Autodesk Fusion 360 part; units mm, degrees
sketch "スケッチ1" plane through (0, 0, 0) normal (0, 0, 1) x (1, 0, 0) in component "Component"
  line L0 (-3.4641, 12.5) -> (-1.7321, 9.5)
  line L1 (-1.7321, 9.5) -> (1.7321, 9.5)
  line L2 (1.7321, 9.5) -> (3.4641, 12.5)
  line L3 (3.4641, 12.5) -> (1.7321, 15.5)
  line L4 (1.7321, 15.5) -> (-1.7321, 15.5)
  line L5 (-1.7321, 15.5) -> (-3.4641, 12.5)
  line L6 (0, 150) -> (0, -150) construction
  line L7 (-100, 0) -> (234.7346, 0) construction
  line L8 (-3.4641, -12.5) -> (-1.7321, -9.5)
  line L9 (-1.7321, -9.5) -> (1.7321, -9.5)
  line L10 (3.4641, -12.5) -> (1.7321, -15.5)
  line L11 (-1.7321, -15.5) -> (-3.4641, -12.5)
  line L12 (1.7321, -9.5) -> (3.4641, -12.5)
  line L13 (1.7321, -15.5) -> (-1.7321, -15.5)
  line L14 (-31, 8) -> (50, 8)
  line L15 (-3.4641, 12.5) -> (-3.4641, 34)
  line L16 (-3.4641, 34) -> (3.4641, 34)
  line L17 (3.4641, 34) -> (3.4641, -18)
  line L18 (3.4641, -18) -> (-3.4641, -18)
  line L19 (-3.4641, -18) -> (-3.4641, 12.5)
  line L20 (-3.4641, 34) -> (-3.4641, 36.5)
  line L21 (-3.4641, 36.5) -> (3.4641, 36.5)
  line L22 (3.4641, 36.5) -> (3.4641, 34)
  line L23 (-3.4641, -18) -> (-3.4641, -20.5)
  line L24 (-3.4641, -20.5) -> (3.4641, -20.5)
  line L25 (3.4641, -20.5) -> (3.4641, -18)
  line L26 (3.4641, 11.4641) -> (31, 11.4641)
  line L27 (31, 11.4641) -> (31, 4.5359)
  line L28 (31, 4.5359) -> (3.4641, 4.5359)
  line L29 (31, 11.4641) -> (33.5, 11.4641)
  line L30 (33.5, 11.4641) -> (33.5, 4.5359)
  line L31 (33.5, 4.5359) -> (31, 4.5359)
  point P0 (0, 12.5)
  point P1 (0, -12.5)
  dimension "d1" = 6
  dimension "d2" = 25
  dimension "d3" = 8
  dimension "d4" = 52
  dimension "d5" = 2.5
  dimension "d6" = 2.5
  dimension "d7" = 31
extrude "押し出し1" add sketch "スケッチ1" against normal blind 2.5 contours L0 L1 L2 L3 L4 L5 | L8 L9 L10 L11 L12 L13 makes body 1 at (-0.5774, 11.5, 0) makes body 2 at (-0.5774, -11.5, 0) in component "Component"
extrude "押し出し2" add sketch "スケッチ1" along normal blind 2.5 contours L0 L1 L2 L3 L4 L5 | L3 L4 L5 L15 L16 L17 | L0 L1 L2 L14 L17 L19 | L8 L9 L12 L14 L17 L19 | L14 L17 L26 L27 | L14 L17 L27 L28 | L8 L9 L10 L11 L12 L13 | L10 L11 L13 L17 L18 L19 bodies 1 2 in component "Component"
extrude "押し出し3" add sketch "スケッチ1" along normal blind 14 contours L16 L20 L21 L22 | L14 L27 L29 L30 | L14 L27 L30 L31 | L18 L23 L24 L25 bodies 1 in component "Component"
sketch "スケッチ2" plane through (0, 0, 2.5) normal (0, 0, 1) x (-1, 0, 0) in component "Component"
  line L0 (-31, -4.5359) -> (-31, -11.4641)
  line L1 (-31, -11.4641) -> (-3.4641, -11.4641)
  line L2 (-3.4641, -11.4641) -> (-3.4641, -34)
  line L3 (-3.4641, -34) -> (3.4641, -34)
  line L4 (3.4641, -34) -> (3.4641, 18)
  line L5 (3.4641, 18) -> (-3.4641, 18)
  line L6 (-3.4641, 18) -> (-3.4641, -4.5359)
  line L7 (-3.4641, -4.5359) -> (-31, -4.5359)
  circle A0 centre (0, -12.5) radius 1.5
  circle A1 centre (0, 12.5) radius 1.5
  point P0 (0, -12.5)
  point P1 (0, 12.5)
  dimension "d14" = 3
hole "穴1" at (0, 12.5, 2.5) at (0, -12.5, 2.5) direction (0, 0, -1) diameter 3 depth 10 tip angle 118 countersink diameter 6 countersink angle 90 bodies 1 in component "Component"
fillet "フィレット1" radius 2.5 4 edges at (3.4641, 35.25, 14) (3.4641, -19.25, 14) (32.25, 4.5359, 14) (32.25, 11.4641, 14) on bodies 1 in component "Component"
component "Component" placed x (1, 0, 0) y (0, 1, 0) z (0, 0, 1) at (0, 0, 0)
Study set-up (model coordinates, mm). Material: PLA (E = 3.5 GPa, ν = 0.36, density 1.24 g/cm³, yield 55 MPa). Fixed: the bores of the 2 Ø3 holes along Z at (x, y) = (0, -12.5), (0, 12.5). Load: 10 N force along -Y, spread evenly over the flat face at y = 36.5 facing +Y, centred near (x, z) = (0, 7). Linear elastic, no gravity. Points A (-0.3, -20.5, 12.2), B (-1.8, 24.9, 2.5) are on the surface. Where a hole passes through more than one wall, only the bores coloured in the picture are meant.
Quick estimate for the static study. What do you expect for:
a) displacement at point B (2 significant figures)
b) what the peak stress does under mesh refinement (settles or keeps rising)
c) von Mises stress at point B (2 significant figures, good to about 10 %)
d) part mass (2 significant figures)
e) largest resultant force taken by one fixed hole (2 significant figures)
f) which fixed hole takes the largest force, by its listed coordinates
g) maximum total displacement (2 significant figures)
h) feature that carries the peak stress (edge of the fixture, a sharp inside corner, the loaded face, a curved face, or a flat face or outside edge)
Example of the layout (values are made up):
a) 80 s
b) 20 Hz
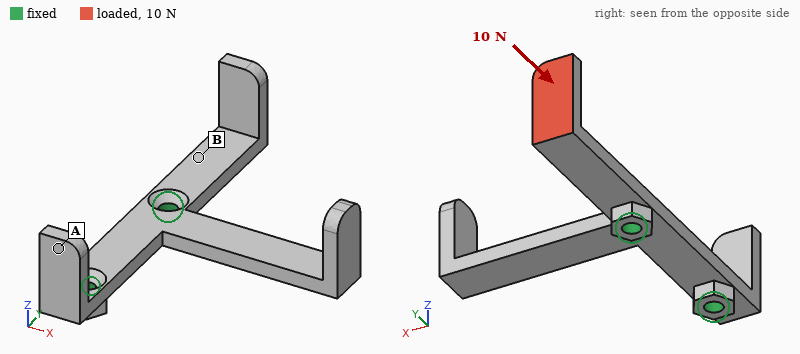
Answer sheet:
a) 0.13 mm
b) keeps rising
c) 8.4 MPa
d) 2.7 g
e) 8.2 N
f) (0, 12.5)
g) 0.75 mm
h) edge of the fixture
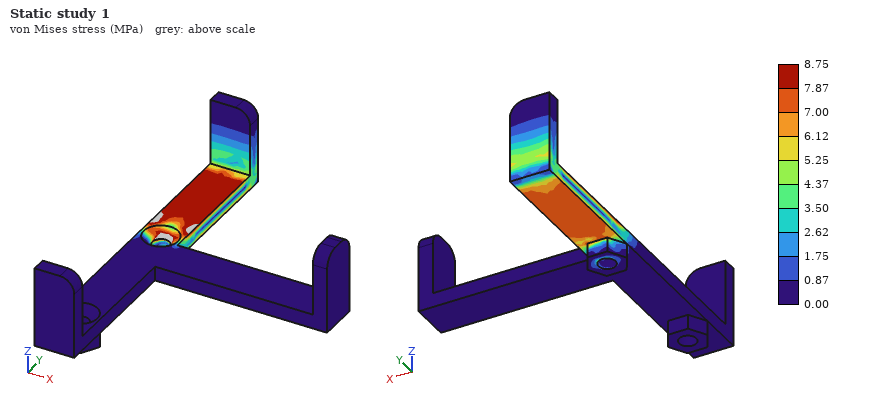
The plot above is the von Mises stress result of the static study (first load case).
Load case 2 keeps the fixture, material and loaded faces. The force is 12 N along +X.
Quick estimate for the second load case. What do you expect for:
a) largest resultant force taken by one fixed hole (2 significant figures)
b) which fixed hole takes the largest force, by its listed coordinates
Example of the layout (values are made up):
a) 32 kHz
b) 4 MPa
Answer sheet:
a) 15 N
b) (0, 12.5)
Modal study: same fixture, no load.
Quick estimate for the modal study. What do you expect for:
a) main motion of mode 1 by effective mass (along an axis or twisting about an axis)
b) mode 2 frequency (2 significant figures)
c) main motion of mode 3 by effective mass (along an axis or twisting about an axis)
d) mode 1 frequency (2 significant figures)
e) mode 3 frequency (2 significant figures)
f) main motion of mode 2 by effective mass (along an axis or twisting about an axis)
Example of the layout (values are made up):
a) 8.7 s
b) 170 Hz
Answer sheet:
a) along Z
b) 700 Hz
c) along Y
d) 390 Hz
e) 940 Hz
f) along Z
